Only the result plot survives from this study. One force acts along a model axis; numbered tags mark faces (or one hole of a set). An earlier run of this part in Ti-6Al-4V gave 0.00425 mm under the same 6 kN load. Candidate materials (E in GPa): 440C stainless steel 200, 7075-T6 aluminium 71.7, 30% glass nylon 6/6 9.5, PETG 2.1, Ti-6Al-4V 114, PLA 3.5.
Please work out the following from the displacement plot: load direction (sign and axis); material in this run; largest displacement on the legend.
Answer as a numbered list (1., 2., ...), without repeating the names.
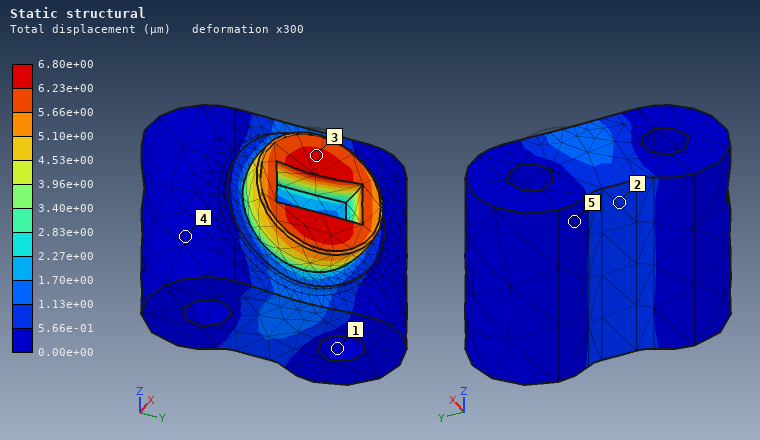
1. -X
2. 7075-T6 aluminium
3. 6.80e+00 µm
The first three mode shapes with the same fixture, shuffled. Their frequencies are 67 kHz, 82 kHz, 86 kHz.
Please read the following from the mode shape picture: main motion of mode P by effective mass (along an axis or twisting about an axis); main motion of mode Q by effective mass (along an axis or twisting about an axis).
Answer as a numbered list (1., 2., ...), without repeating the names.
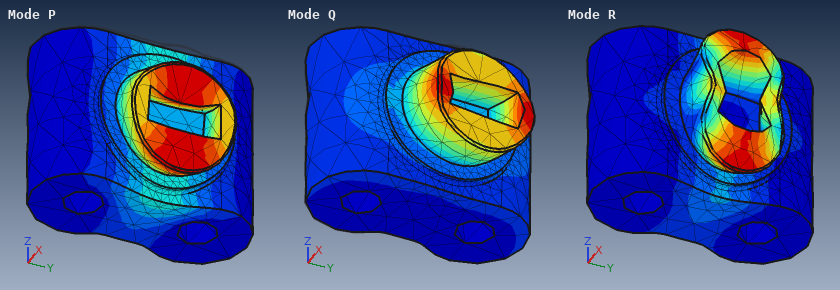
1. along Z
2. along Y
